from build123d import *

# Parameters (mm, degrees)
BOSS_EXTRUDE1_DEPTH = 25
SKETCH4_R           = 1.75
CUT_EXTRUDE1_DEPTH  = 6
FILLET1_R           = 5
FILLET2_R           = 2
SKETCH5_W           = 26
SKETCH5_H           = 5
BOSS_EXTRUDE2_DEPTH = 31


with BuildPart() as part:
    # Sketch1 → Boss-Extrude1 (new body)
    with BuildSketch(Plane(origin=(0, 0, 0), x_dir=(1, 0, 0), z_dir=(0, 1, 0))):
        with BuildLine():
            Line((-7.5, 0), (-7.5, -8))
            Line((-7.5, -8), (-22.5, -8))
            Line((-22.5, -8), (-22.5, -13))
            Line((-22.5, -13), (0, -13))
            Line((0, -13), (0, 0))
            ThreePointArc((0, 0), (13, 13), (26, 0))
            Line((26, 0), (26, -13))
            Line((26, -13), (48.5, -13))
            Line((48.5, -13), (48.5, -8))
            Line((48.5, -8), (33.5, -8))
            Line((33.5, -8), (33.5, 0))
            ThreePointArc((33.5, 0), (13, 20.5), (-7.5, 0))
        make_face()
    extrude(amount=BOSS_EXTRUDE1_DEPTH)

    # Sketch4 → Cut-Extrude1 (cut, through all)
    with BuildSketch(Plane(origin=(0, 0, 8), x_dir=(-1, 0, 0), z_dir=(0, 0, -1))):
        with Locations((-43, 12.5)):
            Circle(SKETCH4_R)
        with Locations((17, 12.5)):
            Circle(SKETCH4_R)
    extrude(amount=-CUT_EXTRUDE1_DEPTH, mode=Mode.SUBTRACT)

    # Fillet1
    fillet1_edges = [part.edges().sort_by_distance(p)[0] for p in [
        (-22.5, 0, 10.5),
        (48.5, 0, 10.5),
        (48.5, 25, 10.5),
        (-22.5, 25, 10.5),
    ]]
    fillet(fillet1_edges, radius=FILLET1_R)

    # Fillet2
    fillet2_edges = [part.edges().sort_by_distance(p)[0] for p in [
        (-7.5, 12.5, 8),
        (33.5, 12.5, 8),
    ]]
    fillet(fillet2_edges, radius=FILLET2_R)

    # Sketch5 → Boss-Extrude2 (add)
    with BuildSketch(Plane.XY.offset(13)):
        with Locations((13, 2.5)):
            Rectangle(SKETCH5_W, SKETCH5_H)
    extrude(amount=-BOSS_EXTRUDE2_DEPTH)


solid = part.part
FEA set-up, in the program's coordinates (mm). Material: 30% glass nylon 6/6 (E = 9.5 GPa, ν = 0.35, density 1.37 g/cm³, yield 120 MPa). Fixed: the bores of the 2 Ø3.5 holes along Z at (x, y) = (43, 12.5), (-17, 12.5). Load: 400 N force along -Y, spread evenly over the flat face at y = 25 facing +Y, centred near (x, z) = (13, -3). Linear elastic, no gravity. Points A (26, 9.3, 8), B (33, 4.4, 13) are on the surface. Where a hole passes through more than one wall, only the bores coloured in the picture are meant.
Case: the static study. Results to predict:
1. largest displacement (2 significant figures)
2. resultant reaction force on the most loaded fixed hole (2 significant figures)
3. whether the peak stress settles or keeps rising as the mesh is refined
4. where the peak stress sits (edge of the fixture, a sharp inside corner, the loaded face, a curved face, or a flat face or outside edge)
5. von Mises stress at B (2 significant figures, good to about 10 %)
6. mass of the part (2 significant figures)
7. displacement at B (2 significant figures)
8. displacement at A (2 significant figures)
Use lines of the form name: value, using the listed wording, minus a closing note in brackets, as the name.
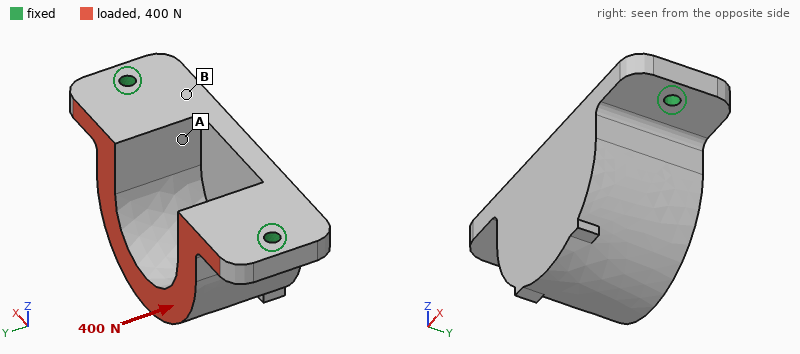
largest displacement: 0.32 mm
resultant reaction force on the most loaded fixed hole: 250 N
whether the peak stress settles or keeps rising as the mesh is refined: keeps rising
where the peak stress sits: edge of the fixture
von Mises stress at B: 11 MPa
mass of the part: 29 g
displacement at B: 0.065 mm
displacement at A: 0.053 mm
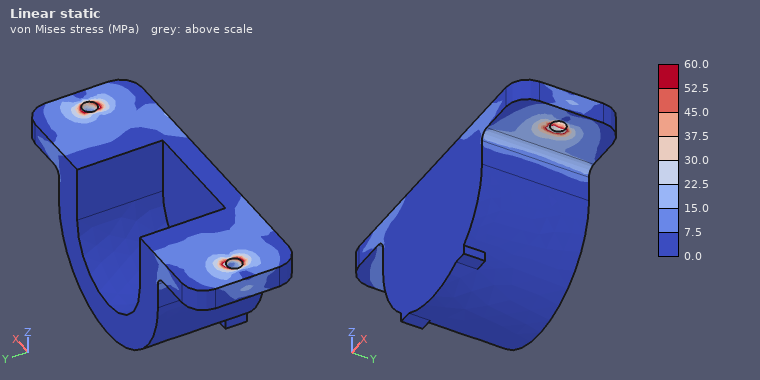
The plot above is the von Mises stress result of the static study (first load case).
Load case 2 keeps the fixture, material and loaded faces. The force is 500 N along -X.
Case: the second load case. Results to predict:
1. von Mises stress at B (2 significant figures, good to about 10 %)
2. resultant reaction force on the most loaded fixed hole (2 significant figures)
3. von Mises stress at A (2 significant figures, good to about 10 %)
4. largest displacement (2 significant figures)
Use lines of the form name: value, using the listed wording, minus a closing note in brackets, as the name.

von Mises stress at B: 4.8 MPa
resultant reaction force on the most loaded fixed hole: 290 N
von Mises stress at A: 3.5 MPa
largest displacement: 68 µm
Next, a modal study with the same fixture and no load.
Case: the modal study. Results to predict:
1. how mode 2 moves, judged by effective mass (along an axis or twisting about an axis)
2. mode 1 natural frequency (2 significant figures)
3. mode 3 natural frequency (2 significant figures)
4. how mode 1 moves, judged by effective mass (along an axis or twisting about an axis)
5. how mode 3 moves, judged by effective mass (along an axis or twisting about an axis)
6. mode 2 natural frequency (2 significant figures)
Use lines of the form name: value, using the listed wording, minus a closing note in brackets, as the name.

how mode 2 moves, judged by effective mass: along Z
mode 1 natural frequency: 1300 Hz
mode 3 natural frequency: 4400 Hz
how mode 1 moves, judged by effective mass: along Y
how mode 3 moves, judged by effective mass: along X
mode 2 natural frequency: 3900 Hz
